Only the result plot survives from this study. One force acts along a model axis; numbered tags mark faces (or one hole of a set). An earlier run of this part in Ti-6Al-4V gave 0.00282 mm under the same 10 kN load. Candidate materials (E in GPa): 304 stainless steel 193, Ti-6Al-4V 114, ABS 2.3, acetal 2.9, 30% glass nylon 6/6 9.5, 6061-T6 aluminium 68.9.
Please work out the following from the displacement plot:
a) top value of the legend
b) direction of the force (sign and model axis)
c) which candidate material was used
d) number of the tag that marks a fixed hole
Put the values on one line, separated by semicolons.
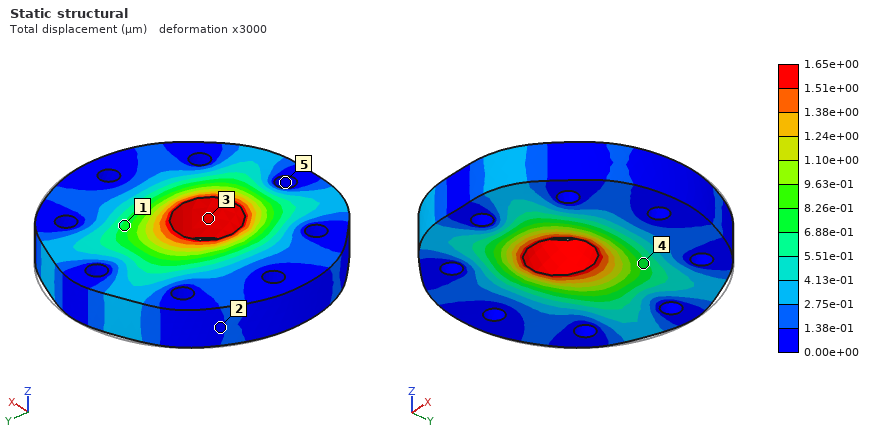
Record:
1.65e+00 µm; -Y; 304 stainless steel; 5
